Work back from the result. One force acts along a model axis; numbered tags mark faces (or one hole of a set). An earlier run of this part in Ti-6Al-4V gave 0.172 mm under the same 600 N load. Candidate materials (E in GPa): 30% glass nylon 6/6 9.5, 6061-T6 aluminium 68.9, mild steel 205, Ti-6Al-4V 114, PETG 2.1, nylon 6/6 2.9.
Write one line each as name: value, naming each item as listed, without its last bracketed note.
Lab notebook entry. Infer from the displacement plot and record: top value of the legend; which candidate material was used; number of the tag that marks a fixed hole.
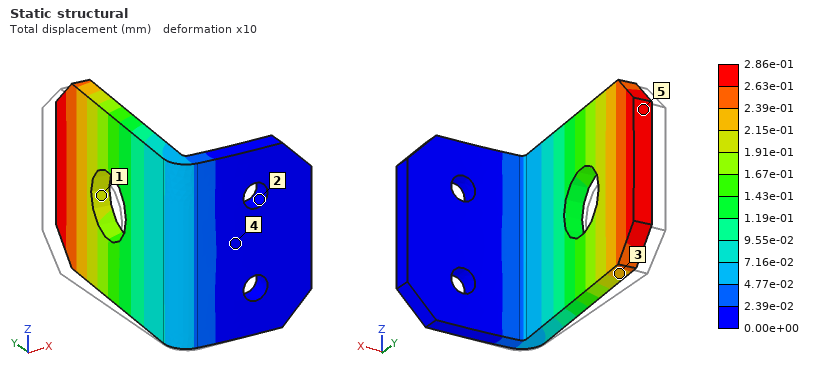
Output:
top value of the legend: 2.86e-01 mm
which candidate material was used: 6061-T6 aluminium
number of the tag that marks a fixed hole: 2
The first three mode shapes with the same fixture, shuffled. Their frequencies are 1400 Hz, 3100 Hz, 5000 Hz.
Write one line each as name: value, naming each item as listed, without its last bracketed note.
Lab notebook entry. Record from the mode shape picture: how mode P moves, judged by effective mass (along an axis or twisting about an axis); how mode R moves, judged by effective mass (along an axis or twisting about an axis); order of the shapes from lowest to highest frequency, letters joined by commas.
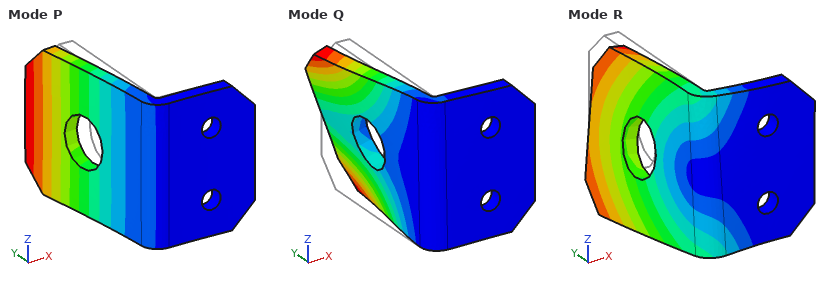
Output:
how mode P moves, judged by effective mass: along X
how mode R moves, judged by effective mass: along Z
order of the shapes from lowest to highest frequency, letters joined by commas: P, R, Q
